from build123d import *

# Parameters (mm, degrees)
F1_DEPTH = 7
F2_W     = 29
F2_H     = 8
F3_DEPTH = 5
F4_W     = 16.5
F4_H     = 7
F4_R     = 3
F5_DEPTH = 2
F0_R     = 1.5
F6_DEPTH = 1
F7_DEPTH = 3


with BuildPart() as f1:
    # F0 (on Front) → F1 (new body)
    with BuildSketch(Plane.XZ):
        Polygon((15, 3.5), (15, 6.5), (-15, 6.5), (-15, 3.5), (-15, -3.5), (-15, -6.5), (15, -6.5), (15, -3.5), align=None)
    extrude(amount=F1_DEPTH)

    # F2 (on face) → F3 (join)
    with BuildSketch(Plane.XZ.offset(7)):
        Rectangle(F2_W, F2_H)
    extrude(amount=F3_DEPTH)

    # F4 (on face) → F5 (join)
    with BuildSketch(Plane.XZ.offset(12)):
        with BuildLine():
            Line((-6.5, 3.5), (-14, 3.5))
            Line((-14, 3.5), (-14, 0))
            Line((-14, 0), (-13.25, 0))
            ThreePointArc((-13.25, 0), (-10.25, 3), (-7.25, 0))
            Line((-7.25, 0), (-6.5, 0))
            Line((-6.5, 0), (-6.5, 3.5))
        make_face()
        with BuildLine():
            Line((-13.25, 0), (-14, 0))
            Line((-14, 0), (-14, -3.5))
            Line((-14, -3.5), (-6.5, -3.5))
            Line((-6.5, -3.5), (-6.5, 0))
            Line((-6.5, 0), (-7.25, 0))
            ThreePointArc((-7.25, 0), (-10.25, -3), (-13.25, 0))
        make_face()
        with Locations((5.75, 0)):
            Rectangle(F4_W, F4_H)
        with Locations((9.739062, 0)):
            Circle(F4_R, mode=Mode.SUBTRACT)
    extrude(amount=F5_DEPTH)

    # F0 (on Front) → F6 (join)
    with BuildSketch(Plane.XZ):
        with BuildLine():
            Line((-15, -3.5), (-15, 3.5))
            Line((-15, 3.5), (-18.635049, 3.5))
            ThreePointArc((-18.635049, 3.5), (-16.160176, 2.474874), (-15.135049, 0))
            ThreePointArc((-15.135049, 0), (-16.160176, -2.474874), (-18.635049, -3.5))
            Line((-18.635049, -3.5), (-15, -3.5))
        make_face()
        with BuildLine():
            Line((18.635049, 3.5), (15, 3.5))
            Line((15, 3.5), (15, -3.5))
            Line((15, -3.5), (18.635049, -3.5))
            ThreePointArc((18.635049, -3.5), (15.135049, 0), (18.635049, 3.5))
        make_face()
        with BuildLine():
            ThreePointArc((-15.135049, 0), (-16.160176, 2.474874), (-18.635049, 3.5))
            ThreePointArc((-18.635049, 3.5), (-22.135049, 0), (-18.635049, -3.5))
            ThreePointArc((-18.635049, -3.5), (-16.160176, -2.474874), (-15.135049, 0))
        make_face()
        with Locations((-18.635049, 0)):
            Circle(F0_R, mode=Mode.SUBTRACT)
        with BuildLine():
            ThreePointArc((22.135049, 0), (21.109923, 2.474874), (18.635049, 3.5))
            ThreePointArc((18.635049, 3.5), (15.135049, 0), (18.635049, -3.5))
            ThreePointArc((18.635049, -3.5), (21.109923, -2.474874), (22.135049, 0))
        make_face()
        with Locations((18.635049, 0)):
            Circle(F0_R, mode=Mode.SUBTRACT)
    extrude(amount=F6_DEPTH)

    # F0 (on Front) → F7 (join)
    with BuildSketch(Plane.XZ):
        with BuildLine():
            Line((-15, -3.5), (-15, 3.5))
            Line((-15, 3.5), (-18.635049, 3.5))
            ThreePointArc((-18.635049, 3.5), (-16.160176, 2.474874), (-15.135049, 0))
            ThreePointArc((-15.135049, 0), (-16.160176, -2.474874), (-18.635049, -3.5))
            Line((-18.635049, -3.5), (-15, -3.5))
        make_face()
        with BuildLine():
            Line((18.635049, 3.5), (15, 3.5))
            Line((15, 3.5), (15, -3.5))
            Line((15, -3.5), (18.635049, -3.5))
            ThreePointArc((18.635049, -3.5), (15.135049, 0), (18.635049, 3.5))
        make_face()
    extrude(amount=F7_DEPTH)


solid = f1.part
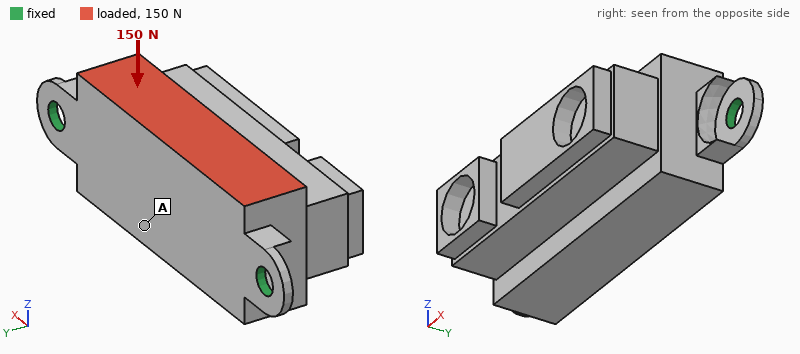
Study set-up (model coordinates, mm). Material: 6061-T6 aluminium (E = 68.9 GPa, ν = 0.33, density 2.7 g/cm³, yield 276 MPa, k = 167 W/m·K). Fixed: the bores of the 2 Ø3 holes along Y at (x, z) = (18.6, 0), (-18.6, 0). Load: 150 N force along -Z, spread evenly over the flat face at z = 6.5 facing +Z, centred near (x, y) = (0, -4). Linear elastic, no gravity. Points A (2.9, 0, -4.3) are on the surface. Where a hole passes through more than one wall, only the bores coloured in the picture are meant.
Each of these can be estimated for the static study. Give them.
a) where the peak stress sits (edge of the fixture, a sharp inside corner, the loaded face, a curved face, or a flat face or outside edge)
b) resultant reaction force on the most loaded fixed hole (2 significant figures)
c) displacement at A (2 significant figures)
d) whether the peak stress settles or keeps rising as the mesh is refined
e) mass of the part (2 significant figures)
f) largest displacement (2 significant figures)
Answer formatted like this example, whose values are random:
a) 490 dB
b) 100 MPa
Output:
a) edge of the fixture
b) 75 N
c) 11 µm
d) keeps rising
e) 11 g
f) 39 µm
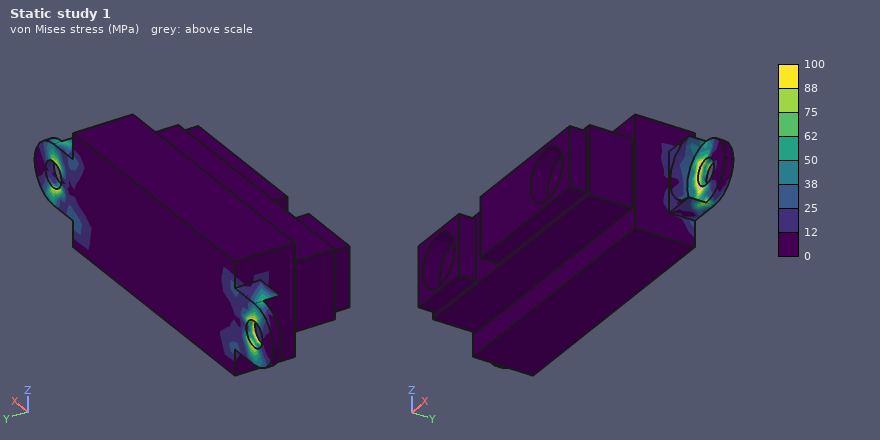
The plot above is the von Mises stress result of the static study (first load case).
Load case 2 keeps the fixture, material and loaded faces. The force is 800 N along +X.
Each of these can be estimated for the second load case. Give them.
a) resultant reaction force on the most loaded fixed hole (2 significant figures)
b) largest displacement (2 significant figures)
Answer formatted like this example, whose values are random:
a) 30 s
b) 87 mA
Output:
a) 430 N
b) 8.1 µm
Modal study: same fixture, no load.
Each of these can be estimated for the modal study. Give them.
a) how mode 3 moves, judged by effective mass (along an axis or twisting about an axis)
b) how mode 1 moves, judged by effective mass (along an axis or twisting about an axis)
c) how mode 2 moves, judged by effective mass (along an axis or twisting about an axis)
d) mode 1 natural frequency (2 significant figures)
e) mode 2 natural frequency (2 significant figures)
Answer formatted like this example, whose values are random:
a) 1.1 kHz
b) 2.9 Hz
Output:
a) along X
b) along Z
c) along Y
d) 2700 Hz
e) 9300 Hz
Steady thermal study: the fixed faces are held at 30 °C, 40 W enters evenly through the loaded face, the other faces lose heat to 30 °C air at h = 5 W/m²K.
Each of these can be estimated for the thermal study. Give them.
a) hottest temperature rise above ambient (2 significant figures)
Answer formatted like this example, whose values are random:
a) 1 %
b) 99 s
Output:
a) 66 K
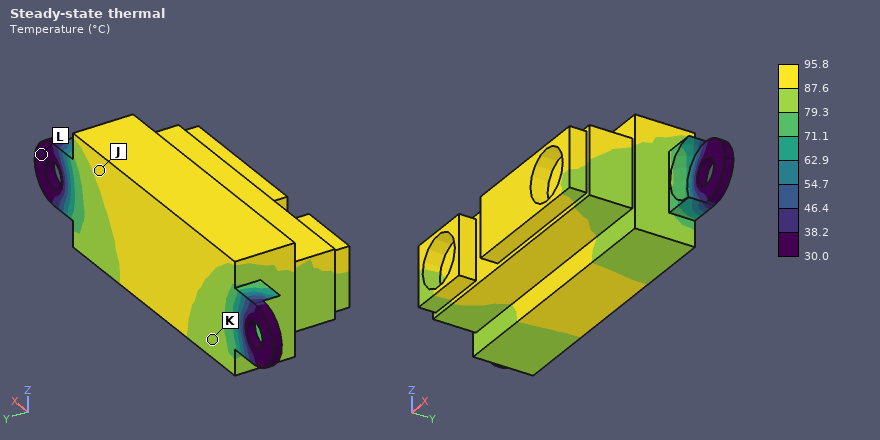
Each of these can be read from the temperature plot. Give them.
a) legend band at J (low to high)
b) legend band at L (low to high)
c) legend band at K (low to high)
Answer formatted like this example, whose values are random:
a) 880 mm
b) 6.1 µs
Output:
a) 87.6 to 95.8 °C
b) 30.0 to 38.2 °C
c) 79.3 to 87.6 °C
